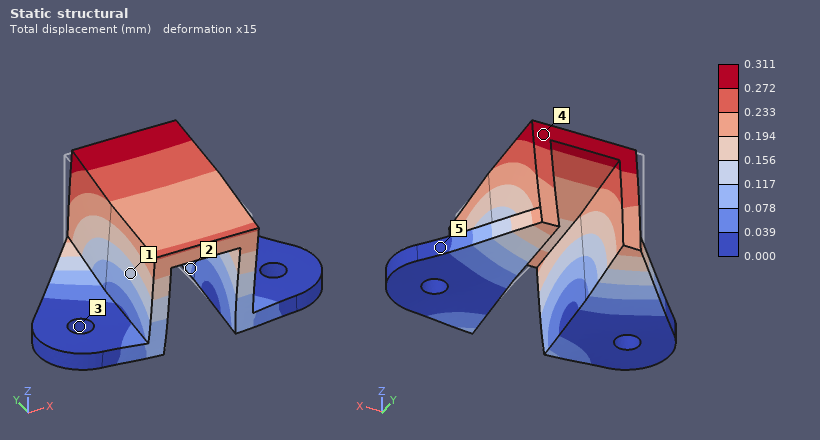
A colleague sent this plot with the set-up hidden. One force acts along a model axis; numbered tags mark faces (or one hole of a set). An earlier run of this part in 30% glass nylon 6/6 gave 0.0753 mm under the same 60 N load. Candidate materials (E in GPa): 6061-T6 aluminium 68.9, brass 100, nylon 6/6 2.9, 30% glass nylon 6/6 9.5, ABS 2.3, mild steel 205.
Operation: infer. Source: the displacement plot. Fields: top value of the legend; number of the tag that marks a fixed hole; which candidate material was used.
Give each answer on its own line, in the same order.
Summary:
0.311 mm
3
ABS
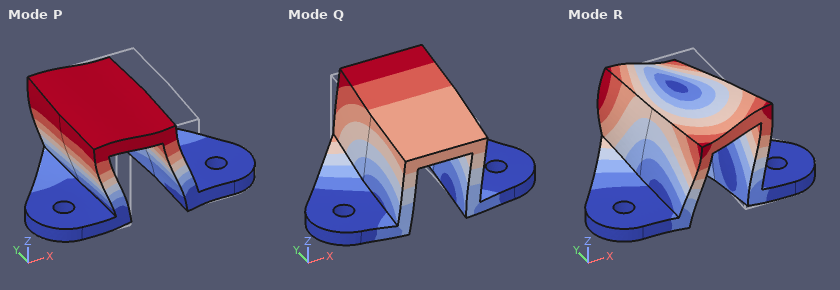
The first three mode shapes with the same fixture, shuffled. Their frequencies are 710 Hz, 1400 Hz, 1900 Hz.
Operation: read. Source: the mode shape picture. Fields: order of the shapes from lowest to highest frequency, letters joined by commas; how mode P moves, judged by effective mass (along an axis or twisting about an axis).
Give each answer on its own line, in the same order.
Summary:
Q, P, R
along X
